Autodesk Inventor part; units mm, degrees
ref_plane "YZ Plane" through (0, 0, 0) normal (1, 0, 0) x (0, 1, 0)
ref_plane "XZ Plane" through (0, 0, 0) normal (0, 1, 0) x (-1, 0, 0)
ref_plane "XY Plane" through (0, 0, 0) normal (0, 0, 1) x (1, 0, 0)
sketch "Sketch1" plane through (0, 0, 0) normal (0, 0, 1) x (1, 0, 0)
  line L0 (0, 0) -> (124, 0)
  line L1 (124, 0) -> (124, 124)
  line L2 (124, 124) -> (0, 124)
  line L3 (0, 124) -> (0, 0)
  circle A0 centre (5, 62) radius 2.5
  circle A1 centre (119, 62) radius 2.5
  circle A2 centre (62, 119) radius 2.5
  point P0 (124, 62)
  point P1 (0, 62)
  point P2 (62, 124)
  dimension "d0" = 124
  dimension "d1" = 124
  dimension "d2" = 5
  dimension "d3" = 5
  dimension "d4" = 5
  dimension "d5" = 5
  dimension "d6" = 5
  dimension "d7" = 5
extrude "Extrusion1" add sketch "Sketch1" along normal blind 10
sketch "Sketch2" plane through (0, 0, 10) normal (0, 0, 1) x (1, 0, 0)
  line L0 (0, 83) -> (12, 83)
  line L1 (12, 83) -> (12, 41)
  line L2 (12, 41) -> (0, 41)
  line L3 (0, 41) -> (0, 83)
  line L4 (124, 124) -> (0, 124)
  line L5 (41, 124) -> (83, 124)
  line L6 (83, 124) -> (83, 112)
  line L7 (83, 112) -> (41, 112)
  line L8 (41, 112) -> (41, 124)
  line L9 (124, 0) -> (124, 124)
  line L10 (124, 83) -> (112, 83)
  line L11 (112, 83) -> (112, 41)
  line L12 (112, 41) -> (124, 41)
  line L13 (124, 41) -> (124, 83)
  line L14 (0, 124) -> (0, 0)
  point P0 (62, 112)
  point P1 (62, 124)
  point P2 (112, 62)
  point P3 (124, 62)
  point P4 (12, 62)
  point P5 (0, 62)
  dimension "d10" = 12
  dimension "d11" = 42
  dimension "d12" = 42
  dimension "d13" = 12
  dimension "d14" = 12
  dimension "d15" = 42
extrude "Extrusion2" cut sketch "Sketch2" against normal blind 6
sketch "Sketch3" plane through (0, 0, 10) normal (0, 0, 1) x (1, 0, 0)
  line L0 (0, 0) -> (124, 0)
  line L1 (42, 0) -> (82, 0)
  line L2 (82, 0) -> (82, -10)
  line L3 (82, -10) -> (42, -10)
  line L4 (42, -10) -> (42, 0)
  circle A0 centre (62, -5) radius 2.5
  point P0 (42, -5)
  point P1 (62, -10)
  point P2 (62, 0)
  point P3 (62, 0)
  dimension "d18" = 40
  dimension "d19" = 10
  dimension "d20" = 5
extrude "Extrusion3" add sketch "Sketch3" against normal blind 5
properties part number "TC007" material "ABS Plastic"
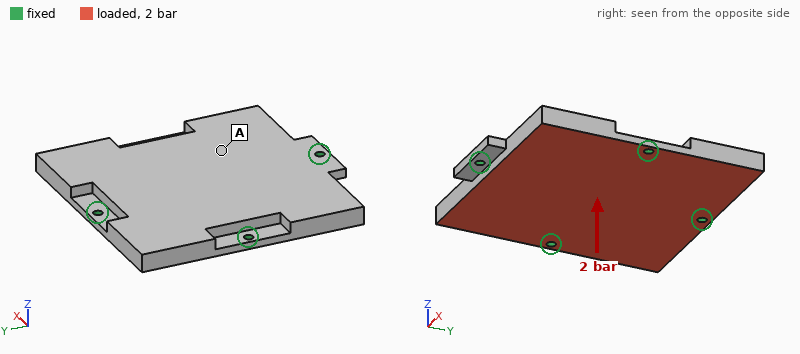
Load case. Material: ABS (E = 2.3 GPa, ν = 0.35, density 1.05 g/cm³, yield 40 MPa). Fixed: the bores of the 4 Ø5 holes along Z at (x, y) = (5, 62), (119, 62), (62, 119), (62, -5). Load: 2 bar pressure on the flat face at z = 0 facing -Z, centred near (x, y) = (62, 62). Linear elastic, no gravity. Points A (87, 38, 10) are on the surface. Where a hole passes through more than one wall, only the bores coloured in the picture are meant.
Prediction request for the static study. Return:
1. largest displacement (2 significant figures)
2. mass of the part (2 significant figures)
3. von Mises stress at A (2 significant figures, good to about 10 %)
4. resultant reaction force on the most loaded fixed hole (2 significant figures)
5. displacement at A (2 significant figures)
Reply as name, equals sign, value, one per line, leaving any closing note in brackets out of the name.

largest displacement = 0.93 mm
mass of the part = 150 g
von Mises stress at A = 6.1 MPa
resultant reaction force on the most loaded fixed hole = 1.0 kN
displacement at A = 0.62 mm
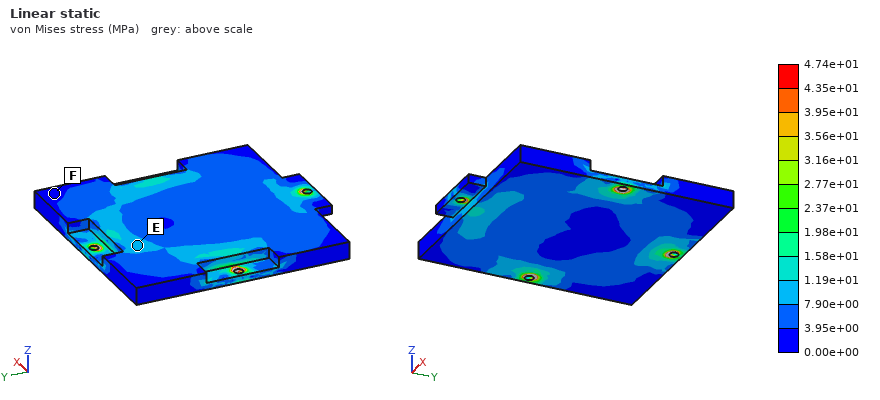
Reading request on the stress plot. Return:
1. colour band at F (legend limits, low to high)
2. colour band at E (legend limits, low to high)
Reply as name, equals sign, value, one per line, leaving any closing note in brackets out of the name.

colour band at F = 0.00e+00 to 3.95e+00 MPa
colour band at E = 7.90e+00 to 1.19e+01 MPa
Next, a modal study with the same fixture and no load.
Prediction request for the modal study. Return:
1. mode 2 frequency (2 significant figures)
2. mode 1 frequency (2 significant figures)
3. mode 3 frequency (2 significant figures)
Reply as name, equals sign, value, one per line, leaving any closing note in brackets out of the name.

mode 2 frequency = 800 Hz
mode 1 frequency = 700 Hz
mode 3 frequency = 800 Hz
